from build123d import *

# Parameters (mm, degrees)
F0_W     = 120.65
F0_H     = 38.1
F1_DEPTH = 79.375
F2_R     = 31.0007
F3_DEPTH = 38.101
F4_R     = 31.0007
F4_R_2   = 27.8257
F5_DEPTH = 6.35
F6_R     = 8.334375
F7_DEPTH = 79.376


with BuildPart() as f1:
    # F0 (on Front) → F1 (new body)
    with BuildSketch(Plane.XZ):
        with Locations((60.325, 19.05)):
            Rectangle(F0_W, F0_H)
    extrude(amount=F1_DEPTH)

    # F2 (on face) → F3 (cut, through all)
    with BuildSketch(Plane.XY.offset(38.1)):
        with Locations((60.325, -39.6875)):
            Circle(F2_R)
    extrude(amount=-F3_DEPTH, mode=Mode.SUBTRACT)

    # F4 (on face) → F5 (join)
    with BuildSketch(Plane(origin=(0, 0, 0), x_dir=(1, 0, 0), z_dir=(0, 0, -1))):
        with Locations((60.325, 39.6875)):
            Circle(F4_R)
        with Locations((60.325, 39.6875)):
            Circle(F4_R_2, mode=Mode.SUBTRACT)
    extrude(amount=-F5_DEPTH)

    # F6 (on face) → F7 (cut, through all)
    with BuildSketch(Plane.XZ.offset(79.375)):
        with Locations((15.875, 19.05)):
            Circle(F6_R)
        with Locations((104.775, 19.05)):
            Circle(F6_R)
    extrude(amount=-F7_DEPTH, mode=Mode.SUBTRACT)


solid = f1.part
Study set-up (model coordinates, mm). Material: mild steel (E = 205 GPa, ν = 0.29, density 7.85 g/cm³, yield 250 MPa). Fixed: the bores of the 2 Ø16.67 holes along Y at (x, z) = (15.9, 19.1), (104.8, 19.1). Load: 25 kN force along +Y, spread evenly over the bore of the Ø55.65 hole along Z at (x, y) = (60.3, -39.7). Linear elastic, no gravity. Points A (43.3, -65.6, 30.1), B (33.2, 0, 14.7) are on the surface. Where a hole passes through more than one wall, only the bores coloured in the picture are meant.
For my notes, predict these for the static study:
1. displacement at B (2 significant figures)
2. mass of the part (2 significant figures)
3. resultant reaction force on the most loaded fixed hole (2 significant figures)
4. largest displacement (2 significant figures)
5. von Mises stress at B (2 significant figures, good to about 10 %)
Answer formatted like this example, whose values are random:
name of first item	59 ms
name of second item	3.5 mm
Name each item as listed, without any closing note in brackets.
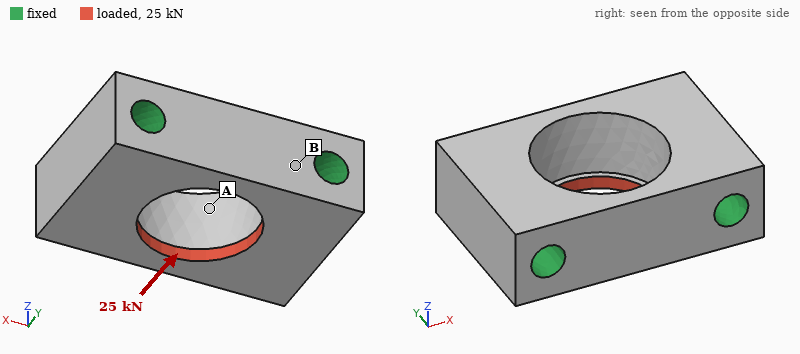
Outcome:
displacement at B	1.8 µm
mass of the part	1.7 kg
resultant reaction force on the most loaded fixed hole	13 kN
largest displacement	12 µm
von Mises stress at B	21 MPa
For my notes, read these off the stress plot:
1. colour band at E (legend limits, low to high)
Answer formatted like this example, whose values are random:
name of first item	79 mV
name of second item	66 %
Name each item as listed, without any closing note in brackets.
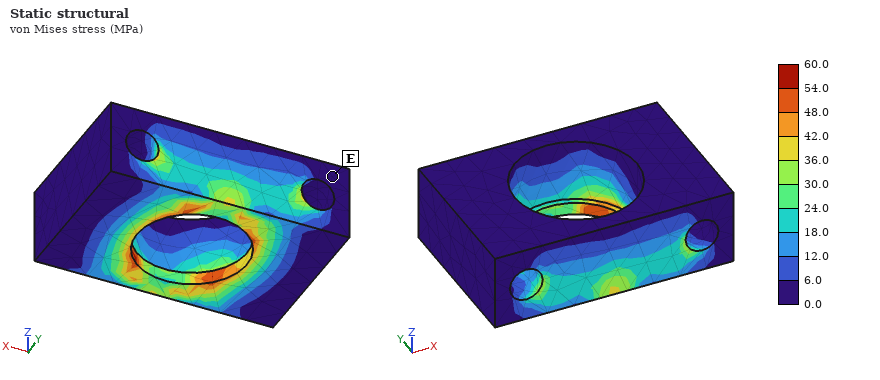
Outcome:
colour band at E	0.0 to 6.0 MPa
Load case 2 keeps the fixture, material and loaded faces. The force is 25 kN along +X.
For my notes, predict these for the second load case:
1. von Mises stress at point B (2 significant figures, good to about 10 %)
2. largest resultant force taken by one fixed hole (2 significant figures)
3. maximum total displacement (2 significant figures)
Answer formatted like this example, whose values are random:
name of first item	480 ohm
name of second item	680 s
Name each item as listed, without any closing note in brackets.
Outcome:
von Mises stress at point B	7.3 MPa
largest resultant force taken by one fixed hole	13 kN
maximum total displacement	3.0 µm
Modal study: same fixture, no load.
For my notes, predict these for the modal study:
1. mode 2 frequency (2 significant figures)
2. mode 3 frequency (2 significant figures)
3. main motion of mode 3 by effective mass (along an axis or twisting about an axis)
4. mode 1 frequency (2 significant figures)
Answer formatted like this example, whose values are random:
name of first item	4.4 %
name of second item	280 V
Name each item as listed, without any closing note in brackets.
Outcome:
mode 2 frequency	17 kHz
mode 3 frequency	18 kHz
main motion of mode 3 by effective mass	along Y
mode 1 frequency	17 kHz
